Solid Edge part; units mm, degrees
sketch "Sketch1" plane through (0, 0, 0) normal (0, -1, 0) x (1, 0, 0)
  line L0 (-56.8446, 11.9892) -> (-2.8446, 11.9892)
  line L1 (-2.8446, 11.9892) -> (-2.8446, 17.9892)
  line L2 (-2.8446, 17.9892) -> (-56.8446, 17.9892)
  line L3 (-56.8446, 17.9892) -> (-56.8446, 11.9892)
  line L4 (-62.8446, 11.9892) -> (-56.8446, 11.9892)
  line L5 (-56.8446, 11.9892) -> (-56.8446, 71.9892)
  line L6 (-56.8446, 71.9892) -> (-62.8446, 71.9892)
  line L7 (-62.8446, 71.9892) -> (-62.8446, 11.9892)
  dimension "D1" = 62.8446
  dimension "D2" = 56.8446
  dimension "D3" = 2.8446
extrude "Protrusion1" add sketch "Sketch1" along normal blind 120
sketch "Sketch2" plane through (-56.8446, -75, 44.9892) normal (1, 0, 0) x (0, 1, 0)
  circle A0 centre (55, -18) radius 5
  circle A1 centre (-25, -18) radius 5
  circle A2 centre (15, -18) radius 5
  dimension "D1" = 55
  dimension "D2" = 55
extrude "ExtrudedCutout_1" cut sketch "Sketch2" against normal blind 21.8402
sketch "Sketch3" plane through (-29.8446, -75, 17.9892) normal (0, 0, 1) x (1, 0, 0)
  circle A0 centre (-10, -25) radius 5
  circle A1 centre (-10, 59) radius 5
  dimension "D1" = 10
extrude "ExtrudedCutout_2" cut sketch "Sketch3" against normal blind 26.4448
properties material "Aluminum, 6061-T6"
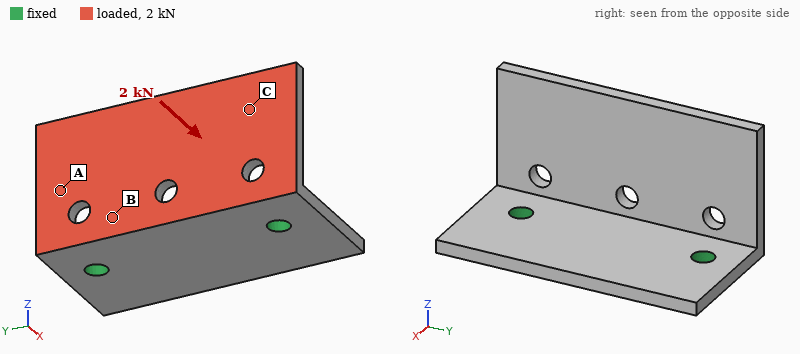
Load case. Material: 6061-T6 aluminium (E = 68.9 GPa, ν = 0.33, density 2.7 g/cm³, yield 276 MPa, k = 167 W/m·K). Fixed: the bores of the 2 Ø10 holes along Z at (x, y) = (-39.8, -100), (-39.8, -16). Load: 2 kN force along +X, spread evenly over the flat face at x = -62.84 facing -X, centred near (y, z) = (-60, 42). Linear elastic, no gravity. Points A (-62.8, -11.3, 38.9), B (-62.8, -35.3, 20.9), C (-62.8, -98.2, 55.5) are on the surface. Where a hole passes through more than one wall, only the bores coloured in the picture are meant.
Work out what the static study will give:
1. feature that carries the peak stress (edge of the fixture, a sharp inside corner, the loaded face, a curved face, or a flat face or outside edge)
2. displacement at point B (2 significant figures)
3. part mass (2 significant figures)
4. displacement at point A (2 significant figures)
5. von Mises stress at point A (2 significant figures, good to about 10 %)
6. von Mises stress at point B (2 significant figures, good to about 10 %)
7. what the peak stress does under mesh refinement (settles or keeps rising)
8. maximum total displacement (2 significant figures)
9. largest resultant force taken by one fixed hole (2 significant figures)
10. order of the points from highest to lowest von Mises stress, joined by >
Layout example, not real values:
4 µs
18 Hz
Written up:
edge of the fixture
0.11 mm
220 g
0.27 mm
28 MPa
62 MPa
keeps rising
0.72 mm
1.0 kN
B > A > C
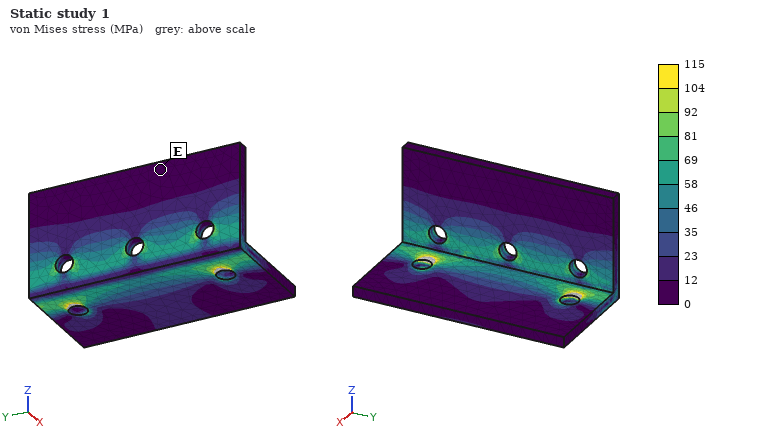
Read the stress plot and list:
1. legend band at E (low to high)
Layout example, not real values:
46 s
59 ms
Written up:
0 to 12 MPa
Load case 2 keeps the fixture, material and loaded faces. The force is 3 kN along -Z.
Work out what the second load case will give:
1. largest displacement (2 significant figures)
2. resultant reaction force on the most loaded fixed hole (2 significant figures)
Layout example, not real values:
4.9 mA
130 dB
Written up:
0.37 mm
1.6 kN
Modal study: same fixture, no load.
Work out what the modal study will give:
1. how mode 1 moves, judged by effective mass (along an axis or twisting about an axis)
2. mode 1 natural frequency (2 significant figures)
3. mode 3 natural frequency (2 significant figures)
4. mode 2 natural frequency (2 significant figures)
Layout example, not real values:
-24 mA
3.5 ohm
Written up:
along X
960 Hz
3000 Hz
1700 Hz
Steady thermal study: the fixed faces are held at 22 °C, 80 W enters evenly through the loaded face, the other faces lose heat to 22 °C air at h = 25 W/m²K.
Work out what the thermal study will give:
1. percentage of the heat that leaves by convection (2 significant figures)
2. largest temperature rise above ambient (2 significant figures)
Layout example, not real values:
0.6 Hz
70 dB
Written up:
11 %
34 K
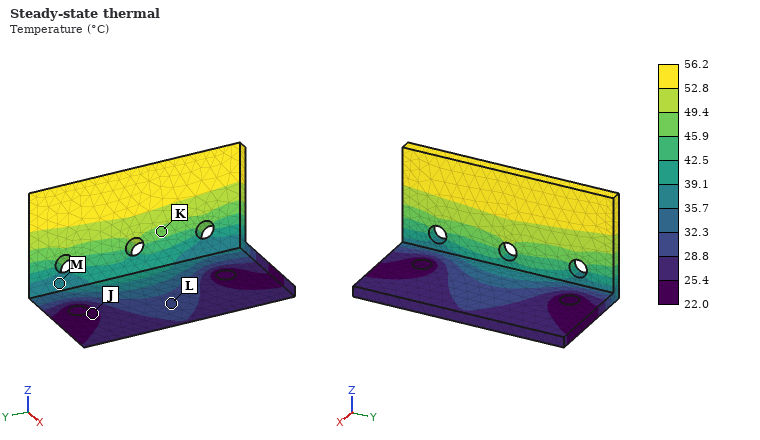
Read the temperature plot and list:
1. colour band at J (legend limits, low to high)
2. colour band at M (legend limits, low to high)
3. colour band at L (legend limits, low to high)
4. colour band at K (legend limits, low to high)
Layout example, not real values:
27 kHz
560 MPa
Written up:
22.0 to 25.4 °C
35.7 to 39.1 °C
28.8 to 32.3 °C
45.9 to 49.4 °C
